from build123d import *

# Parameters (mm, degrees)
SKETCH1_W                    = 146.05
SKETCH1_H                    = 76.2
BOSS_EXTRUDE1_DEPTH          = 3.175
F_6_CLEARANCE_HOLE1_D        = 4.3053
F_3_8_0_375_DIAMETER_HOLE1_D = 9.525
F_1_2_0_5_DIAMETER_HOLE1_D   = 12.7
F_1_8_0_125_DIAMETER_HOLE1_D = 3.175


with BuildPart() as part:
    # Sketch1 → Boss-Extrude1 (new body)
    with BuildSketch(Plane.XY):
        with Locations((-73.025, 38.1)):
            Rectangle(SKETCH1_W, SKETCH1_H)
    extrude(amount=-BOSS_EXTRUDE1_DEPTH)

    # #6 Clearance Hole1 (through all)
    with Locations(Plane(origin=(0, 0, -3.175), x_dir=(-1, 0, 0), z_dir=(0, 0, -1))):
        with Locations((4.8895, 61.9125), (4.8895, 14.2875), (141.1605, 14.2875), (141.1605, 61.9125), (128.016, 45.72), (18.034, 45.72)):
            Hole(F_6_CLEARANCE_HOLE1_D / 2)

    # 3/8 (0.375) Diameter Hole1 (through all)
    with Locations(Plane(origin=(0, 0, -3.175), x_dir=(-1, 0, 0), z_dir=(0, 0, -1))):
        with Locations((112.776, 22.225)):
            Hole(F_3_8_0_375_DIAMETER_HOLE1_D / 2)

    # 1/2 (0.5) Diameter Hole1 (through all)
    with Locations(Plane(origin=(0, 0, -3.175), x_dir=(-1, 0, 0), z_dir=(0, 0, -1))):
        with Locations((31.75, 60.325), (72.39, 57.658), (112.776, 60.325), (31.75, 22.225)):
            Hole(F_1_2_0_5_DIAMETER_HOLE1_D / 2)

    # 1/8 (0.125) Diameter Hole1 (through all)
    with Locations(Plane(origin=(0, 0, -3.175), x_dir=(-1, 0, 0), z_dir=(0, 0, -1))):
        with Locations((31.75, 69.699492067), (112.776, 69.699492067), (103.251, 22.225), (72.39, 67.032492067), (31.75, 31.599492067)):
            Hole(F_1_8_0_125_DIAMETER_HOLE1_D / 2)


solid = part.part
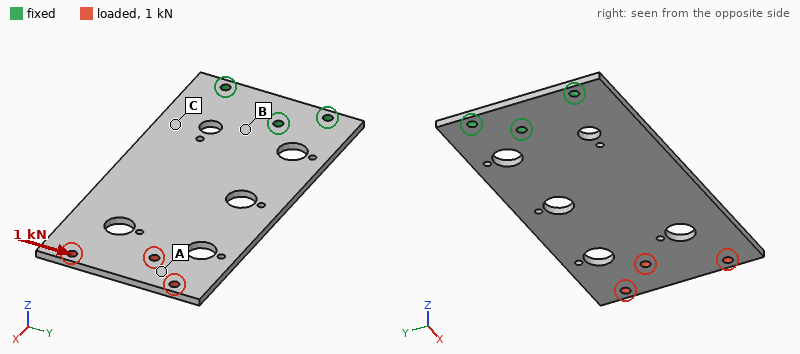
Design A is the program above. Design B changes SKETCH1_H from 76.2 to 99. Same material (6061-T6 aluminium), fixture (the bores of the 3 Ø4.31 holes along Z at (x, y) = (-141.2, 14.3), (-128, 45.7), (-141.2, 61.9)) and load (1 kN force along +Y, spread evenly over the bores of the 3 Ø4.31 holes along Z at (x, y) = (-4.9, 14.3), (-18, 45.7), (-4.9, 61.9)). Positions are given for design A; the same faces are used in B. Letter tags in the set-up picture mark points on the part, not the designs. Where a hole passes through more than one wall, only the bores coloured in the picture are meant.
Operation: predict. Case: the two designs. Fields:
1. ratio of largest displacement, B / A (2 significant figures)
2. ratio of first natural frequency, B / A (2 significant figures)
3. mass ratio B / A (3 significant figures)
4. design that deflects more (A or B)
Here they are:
0.75
0.98
1.32
A
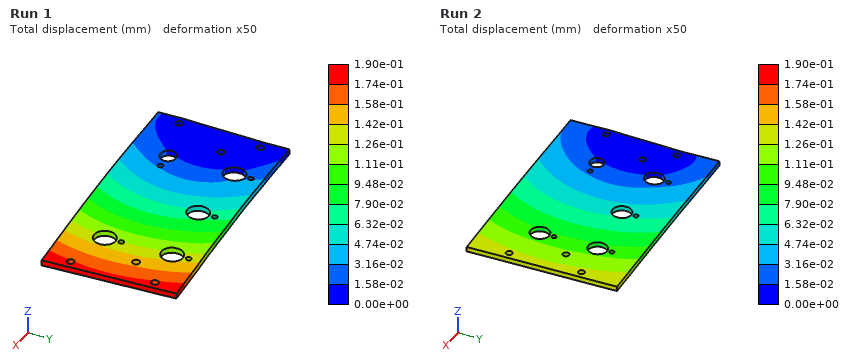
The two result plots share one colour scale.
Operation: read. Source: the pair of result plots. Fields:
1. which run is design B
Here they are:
Run 2
